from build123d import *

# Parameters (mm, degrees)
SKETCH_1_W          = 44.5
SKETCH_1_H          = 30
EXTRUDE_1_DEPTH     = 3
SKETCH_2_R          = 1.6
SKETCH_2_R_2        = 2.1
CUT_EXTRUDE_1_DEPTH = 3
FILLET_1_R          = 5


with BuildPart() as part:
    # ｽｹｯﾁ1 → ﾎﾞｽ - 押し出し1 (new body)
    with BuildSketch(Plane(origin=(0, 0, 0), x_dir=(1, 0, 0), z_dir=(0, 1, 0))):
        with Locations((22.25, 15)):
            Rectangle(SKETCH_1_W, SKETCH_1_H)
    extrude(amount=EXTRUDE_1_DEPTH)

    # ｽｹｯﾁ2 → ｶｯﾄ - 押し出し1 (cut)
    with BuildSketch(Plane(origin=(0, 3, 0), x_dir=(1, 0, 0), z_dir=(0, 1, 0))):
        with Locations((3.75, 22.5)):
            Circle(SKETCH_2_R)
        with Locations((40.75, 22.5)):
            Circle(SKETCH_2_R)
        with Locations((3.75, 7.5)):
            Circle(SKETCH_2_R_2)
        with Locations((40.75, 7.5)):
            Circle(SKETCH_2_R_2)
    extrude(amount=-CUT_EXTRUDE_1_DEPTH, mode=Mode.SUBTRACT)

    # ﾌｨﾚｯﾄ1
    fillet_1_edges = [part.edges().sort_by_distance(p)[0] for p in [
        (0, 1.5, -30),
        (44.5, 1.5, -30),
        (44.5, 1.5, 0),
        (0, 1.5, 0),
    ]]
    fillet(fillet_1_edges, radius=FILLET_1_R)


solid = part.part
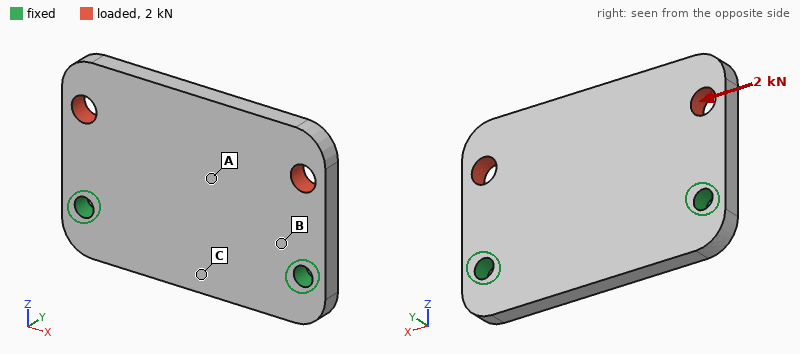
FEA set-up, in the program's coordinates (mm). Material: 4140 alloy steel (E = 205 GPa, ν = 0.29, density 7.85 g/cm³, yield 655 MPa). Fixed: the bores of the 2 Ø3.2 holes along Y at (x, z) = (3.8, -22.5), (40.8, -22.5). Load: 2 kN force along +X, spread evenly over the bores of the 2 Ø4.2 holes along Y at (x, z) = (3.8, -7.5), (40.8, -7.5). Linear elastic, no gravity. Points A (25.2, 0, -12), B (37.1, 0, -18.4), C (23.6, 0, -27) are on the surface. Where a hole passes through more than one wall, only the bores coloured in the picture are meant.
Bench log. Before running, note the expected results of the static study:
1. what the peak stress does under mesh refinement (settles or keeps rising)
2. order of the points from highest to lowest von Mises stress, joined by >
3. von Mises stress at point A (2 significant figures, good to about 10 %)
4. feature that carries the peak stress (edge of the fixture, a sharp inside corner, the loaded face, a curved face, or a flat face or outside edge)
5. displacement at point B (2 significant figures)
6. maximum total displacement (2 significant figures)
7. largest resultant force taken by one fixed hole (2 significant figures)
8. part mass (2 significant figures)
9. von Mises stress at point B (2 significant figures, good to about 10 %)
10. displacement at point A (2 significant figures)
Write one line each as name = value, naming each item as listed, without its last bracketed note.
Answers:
what the peak stress does under mesh refinement = keeps rising
order of the points from highest to lowest von Mises stress, joined by > = B > A > C
von Mises stress at point A = 25 MPa
feature that carries the peak stress = edge of the fixture
displacement at point B = 1.3 µm
maximum total displacement = 6.7 µm
largest resultant force taken by one fixed hole = 1.3 kN
part mass = 30 g
von Mises stress at point B = 43 MPa
displacement at point A = 3.0 µm
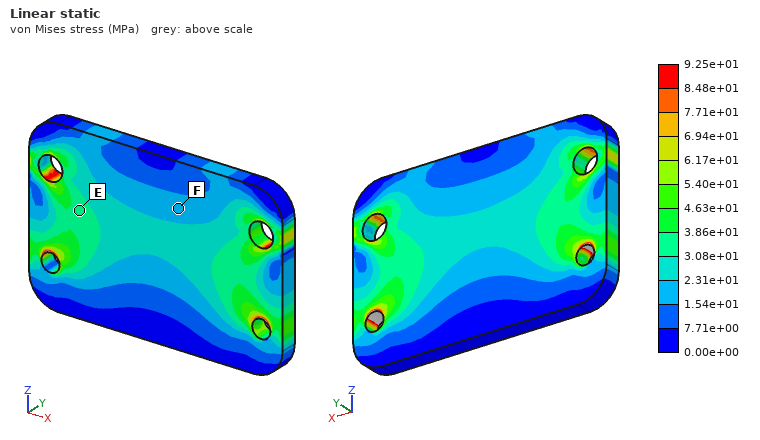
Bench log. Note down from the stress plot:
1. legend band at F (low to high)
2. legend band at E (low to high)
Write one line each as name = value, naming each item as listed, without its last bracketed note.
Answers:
legend band at F = 1.54e+01 to 2.31e+01 MPa
legend band at E = 3.08e+01 to 3.86e+01 MPa
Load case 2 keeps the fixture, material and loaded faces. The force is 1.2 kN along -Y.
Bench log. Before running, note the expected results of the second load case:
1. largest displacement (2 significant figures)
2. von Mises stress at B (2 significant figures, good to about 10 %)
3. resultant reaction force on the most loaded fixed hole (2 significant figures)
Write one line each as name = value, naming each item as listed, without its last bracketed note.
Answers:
largest displacement = 0.16 mm
von Mises stress at B = 220 MPa
resultant reaction force on the most loaded fixed hole = 600 N
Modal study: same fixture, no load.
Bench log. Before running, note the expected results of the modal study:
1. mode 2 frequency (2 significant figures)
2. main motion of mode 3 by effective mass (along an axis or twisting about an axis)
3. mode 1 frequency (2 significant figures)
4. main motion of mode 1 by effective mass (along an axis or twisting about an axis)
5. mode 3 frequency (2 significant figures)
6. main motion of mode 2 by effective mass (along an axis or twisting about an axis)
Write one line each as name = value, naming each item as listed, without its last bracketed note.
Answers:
mode 2 frequency = 8100 Hz
main motion of mode 3 by effective mass = along Y
mode 1 frequency = 3900 Hz
main motion of mode 1 by effective mass = along Y
mode 3 frequency = 11 kHz
main motion of mode 2 by effective mass = twisting about Z
